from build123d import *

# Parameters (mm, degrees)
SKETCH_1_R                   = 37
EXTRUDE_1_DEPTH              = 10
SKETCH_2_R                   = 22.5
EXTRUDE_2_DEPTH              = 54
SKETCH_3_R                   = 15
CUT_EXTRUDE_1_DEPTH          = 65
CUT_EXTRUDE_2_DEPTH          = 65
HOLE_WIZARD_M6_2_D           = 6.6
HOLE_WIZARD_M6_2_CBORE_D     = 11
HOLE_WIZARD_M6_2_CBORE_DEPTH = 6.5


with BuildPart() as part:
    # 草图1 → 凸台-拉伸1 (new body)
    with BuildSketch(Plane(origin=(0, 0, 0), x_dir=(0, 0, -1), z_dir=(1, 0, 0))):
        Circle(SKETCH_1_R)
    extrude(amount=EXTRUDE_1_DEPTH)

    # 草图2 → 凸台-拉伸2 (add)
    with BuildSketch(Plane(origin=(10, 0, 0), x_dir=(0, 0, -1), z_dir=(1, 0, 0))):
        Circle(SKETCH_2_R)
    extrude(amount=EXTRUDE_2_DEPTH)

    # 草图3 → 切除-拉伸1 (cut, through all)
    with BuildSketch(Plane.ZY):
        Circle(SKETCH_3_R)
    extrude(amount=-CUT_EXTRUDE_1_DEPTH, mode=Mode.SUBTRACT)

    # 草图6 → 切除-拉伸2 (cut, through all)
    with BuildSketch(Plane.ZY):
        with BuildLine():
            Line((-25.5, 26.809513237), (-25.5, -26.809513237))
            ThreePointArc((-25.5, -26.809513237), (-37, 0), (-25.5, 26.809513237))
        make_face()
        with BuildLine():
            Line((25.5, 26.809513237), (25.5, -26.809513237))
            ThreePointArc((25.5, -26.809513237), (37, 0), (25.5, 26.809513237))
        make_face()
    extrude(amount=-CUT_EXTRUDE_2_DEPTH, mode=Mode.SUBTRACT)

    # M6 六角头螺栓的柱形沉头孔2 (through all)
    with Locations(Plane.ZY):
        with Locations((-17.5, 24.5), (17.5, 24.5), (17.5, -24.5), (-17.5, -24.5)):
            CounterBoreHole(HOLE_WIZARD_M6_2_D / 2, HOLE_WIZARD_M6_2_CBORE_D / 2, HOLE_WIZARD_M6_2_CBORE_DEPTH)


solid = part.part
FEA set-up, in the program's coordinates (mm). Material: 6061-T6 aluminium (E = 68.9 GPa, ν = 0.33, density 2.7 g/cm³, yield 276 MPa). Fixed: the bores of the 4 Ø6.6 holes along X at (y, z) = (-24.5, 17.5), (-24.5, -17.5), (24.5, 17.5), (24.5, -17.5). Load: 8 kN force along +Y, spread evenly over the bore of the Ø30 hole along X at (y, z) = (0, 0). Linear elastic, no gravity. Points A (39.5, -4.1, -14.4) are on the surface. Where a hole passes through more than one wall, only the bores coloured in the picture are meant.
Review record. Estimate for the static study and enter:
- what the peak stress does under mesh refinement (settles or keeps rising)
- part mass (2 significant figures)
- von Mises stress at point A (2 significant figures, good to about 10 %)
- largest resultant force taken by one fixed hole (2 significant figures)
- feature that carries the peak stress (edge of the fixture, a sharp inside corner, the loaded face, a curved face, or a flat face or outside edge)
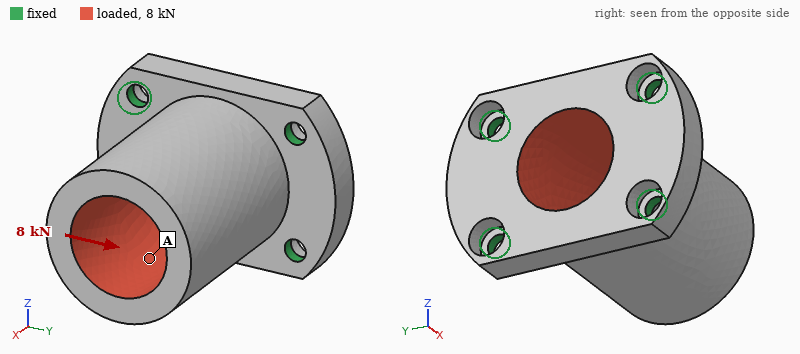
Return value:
keeps rising
190 g
14 MPa
2.9 kN
edge of the fixture
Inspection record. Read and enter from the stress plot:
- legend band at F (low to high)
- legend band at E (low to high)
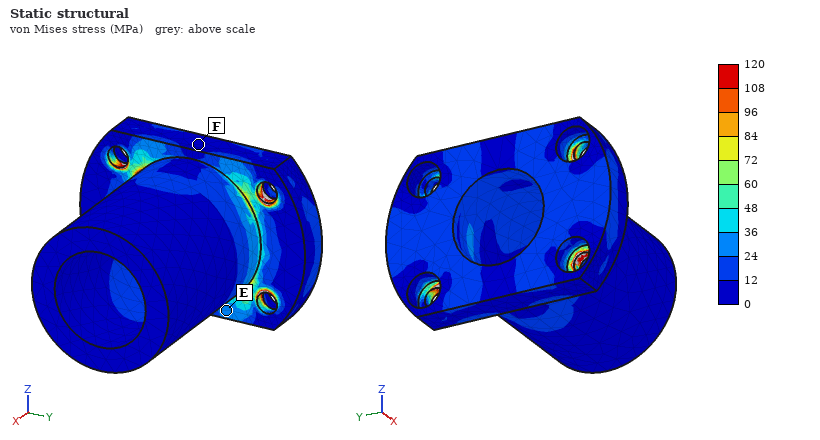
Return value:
0 to 12 MPa
24 to 36 MPa
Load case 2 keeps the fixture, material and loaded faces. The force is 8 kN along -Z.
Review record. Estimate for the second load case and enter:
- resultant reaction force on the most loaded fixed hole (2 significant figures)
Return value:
3.4 kN
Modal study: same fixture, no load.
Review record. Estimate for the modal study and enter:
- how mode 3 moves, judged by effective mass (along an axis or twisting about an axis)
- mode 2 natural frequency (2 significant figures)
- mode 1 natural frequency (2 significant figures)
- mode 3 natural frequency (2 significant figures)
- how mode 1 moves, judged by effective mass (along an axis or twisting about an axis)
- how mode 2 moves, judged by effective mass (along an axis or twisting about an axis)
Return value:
along X
5100 Hz
4000 Hz
8700 Hz
along Z
along Y
